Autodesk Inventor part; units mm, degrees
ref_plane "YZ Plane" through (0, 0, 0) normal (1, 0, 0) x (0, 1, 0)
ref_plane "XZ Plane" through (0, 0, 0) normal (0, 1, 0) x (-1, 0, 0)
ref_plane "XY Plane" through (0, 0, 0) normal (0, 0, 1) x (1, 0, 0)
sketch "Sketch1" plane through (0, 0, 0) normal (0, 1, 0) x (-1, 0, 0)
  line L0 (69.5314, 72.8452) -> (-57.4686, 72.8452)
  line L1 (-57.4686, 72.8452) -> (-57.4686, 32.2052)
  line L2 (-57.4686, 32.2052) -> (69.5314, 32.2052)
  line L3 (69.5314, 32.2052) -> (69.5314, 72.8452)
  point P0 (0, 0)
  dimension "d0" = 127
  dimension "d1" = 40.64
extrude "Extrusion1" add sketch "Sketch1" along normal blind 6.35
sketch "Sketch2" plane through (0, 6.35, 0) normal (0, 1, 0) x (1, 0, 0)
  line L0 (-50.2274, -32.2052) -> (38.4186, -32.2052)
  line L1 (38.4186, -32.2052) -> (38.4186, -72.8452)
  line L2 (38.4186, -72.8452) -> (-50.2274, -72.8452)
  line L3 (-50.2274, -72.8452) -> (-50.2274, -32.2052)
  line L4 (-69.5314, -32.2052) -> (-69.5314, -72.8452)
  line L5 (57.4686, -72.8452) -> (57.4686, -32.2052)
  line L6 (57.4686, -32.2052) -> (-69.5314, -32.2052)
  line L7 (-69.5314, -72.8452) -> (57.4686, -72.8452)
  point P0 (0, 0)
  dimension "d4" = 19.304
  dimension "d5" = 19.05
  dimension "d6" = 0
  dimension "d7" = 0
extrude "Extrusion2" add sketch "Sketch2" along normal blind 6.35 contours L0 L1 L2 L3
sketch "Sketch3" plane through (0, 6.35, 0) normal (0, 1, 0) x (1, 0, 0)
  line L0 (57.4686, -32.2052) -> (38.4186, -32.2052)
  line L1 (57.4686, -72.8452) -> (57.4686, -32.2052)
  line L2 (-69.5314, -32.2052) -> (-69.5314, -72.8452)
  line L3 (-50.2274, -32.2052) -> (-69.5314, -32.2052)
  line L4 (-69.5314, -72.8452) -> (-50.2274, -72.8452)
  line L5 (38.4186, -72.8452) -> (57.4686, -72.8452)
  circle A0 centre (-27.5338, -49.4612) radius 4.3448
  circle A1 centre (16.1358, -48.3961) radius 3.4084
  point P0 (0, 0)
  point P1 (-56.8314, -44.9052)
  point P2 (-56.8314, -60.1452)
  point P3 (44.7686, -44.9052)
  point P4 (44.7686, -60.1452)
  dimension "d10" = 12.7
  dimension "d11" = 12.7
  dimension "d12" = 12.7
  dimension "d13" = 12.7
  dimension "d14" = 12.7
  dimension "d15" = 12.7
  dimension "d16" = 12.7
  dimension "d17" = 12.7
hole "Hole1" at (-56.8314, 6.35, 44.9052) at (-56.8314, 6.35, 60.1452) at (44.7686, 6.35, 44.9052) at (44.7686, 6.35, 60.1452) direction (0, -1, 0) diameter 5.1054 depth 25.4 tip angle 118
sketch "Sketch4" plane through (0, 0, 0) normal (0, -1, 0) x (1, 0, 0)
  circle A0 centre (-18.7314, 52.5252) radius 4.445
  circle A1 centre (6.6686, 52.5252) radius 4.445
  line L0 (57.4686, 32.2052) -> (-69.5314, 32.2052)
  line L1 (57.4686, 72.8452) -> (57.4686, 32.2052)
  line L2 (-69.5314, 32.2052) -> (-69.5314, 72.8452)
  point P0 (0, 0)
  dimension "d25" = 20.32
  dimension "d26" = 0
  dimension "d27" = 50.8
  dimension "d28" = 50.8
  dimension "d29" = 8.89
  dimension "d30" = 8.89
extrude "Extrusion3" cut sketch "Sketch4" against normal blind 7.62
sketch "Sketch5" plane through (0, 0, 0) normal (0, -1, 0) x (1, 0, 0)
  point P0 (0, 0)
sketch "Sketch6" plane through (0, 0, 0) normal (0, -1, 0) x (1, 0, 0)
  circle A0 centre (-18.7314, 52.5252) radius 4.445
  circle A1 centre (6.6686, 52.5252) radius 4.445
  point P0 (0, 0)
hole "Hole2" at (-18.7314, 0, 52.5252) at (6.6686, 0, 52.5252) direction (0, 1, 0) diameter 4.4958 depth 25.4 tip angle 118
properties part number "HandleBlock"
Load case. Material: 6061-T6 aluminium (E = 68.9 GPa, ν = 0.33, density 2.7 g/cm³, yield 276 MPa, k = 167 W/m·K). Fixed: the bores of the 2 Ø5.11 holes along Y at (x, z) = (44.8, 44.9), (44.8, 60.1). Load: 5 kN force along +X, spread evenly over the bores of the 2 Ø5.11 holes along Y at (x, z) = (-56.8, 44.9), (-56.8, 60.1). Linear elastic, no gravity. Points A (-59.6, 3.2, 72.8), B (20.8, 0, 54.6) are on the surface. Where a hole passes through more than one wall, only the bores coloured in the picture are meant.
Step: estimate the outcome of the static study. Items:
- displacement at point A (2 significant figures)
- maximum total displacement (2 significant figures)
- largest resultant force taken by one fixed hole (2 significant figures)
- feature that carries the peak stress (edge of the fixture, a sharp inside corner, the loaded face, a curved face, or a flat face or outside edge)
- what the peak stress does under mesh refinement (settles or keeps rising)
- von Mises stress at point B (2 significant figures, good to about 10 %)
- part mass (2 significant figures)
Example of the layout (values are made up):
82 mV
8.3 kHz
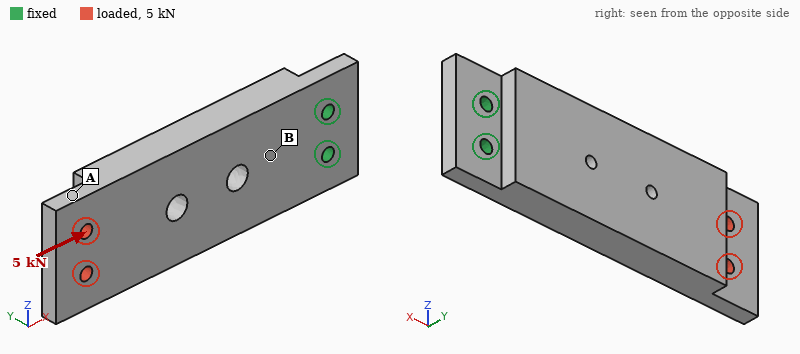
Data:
0.17 mm
0.21 mm
2.5 kN
edge of the fixture
keeps rising
22 MPa
150 g
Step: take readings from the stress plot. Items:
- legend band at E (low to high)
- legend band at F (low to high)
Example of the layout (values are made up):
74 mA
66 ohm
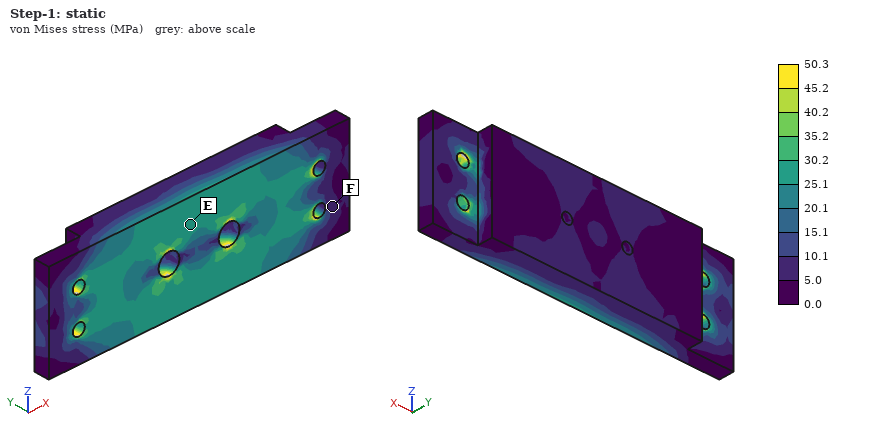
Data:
25.1 to 30.2 MPa
5.0 to 10.1 MPa
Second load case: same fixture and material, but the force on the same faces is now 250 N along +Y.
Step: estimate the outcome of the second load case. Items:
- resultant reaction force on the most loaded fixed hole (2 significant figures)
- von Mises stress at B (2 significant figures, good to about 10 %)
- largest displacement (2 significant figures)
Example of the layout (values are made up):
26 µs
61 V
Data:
130 N
16 MPa
0.57 mm
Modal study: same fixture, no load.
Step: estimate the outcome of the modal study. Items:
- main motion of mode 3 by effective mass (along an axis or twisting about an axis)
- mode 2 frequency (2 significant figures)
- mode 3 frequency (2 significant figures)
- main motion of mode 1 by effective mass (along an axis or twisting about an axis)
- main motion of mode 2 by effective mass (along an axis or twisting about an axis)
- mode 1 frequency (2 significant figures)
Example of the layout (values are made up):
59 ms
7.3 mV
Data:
twisting about X
1800 Hz
3500 Hz
along Y
along Z
530 Hz
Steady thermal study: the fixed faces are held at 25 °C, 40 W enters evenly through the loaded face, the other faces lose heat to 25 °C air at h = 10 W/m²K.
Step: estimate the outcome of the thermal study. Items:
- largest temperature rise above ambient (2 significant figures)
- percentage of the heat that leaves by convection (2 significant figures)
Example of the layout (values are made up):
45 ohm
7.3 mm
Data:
58 K
9.8 %
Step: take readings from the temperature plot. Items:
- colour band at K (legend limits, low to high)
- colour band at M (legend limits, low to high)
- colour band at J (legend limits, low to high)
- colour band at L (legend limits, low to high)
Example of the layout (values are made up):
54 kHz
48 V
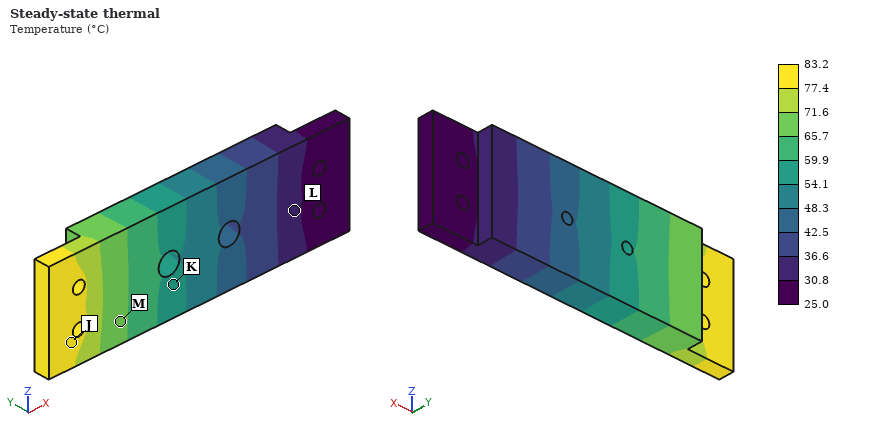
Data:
54.1 to 59.9 °C
65.7 to 71.6 °C
77.4 to 83.2 °C
30.8 to 36.6 °C
